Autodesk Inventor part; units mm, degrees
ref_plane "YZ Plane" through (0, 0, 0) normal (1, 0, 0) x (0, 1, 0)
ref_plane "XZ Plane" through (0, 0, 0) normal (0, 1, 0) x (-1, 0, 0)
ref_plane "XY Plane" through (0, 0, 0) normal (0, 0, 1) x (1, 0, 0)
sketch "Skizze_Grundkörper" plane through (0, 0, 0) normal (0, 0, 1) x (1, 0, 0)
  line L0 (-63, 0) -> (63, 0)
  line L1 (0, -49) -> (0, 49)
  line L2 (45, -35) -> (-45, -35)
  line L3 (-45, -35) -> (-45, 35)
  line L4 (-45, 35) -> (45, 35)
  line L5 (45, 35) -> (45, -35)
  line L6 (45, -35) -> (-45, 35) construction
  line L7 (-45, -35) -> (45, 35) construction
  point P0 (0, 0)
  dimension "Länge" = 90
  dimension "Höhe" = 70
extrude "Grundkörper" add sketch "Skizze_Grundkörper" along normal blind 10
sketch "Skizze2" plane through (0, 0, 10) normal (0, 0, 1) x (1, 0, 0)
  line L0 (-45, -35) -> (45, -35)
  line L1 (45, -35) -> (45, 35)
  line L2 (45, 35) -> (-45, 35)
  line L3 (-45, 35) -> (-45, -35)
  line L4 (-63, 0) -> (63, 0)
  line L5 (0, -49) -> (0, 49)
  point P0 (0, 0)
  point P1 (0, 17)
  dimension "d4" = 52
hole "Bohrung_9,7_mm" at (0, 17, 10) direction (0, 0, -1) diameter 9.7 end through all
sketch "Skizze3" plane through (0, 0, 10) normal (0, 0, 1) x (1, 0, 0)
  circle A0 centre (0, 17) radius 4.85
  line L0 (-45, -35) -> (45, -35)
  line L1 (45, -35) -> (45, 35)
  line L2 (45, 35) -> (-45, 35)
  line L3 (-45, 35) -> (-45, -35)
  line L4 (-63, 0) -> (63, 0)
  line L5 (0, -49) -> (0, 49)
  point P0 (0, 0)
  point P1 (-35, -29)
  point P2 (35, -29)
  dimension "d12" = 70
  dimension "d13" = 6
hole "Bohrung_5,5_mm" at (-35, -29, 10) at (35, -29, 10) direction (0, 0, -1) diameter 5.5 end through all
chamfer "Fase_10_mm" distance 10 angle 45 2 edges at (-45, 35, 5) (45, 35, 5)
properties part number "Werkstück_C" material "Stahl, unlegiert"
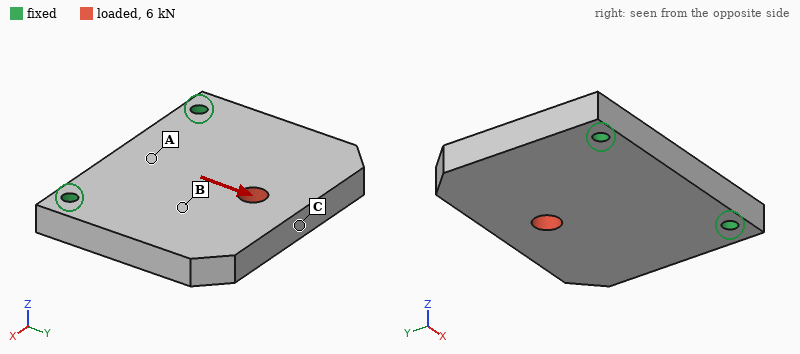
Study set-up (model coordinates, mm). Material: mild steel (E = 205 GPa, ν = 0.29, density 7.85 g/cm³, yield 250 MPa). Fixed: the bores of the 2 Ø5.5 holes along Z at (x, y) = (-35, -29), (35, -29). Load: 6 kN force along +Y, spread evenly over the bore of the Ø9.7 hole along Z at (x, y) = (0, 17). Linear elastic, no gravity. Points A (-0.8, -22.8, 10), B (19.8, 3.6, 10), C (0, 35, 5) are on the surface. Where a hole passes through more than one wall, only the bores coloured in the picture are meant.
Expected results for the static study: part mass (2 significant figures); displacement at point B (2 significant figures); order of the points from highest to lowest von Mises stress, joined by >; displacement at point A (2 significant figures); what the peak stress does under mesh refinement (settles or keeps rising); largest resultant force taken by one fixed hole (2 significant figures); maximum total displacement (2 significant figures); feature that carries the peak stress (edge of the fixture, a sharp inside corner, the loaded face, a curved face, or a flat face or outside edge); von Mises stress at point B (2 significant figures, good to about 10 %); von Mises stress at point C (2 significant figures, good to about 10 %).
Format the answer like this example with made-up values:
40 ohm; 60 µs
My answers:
480 g; 2.5 µm; C > B > A; 2.7 µm; keeps rising; 3.2 kN; 5.1 µm; edge of the fixture; 11 MPa; 22 MPa
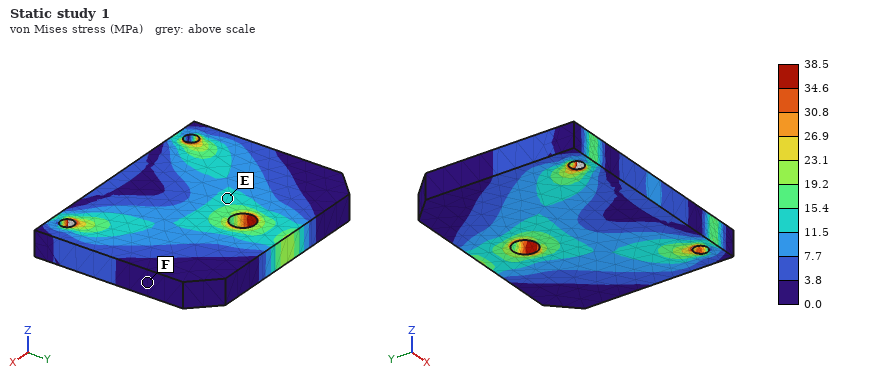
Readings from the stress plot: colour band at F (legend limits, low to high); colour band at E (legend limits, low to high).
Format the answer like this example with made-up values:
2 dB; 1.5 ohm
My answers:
0.0 to 3.8 MPa; 11.5 to 15.4 MPa
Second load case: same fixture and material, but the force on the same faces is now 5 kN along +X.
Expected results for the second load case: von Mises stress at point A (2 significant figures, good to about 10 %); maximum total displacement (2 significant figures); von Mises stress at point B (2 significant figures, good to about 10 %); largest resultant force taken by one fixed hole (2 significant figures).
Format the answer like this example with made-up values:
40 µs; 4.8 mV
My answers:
6.3 MPa; 7.5 µm; 12 MPa; 4.0 kN
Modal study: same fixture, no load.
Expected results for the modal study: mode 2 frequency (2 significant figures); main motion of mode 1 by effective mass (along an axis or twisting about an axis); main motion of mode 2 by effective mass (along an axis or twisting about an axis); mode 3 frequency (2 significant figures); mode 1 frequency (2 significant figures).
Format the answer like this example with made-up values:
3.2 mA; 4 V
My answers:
3800 Hz; along Z; twisting about Y; 7800 Hz; 1600 Hz
